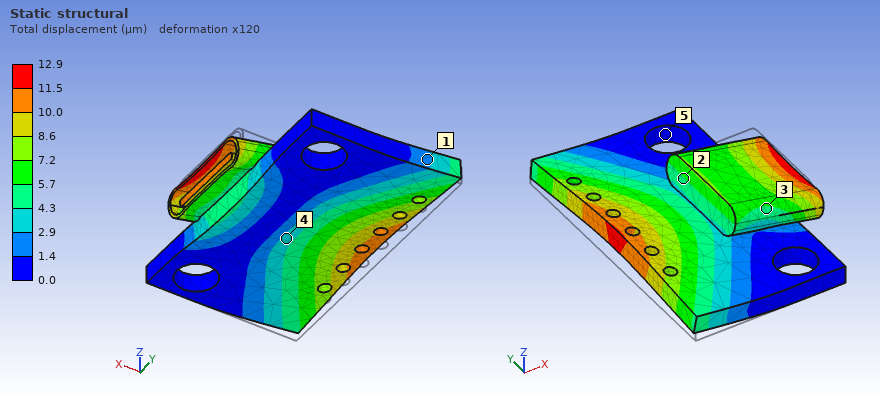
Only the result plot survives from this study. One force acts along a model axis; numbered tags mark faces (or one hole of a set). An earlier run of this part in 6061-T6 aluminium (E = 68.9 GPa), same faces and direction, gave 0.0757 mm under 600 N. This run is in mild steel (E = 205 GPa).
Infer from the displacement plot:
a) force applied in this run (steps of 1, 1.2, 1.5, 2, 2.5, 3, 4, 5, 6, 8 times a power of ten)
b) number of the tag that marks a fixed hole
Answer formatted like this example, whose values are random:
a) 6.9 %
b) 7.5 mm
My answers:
a) 300 N
b) 5
